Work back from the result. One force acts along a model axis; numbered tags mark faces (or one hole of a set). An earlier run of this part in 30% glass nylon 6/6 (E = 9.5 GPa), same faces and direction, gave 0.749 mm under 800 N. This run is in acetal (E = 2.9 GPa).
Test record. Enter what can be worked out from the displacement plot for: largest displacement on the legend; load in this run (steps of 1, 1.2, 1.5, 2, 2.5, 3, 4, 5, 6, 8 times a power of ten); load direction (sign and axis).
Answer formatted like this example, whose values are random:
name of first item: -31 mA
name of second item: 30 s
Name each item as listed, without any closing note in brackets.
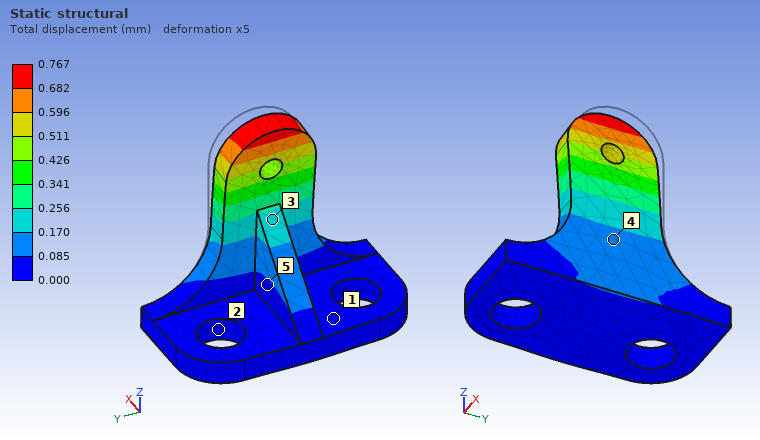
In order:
largest displacement on the legend: 0.767 mm
load in this run: 250 N
load direction: -X
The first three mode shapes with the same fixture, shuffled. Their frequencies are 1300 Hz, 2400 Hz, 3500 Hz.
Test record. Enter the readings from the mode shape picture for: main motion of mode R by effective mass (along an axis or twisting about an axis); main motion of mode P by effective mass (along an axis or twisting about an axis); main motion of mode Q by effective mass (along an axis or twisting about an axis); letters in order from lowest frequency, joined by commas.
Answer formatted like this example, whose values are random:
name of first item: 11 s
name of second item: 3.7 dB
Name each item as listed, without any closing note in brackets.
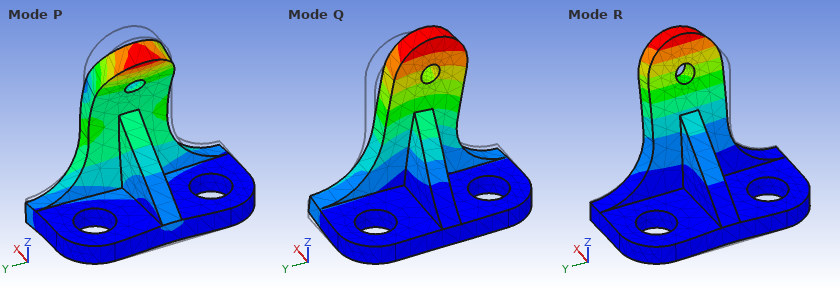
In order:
main motion of mode R by effective mass: along X
main motion of mode P by effective mass: along Z
main motion of mode Q by effective mass: along Y
letters in order from lowest frequency, joined by commas: R, Q, P
